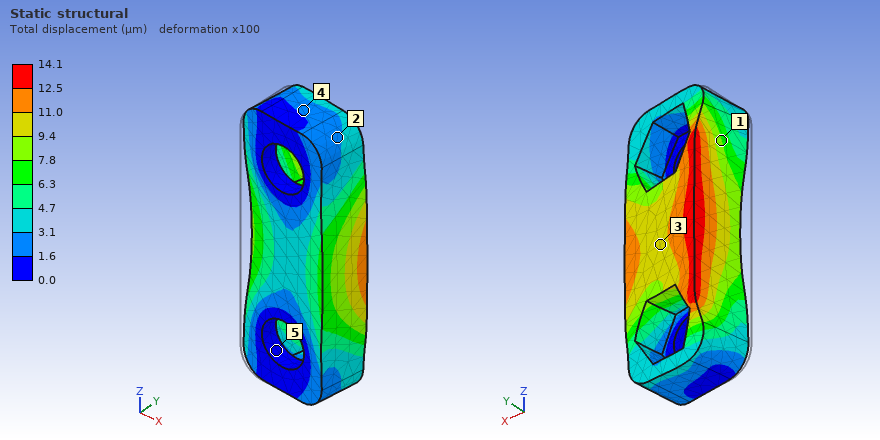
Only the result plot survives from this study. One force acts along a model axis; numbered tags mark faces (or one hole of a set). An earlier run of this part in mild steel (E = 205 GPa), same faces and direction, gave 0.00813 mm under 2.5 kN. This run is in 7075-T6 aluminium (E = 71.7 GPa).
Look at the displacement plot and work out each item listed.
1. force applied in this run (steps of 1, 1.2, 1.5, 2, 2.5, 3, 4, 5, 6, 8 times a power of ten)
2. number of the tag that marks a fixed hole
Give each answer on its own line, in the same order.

1.5 kN
5
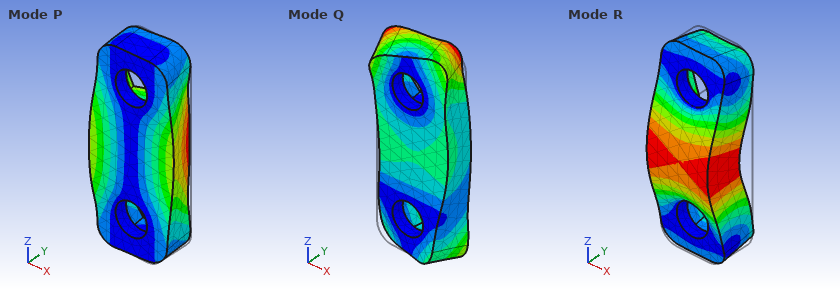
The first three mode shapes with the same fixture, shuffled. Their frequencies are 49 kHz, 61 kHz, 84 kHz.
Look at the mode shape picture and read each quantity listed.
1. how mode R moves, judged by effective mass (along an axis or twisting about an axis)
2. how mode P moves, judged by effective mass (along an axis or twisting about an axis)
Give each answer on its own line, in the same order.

along Y
along X
